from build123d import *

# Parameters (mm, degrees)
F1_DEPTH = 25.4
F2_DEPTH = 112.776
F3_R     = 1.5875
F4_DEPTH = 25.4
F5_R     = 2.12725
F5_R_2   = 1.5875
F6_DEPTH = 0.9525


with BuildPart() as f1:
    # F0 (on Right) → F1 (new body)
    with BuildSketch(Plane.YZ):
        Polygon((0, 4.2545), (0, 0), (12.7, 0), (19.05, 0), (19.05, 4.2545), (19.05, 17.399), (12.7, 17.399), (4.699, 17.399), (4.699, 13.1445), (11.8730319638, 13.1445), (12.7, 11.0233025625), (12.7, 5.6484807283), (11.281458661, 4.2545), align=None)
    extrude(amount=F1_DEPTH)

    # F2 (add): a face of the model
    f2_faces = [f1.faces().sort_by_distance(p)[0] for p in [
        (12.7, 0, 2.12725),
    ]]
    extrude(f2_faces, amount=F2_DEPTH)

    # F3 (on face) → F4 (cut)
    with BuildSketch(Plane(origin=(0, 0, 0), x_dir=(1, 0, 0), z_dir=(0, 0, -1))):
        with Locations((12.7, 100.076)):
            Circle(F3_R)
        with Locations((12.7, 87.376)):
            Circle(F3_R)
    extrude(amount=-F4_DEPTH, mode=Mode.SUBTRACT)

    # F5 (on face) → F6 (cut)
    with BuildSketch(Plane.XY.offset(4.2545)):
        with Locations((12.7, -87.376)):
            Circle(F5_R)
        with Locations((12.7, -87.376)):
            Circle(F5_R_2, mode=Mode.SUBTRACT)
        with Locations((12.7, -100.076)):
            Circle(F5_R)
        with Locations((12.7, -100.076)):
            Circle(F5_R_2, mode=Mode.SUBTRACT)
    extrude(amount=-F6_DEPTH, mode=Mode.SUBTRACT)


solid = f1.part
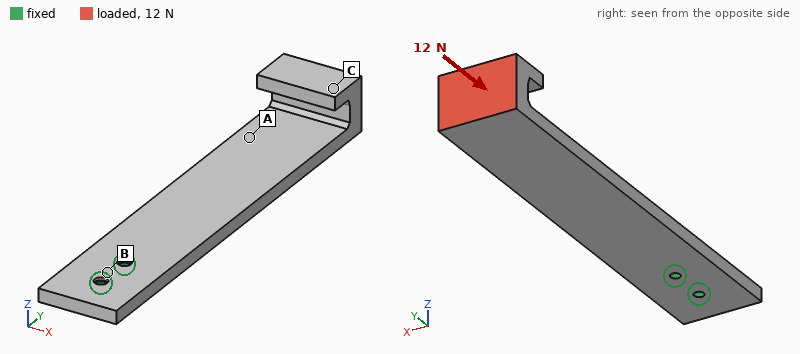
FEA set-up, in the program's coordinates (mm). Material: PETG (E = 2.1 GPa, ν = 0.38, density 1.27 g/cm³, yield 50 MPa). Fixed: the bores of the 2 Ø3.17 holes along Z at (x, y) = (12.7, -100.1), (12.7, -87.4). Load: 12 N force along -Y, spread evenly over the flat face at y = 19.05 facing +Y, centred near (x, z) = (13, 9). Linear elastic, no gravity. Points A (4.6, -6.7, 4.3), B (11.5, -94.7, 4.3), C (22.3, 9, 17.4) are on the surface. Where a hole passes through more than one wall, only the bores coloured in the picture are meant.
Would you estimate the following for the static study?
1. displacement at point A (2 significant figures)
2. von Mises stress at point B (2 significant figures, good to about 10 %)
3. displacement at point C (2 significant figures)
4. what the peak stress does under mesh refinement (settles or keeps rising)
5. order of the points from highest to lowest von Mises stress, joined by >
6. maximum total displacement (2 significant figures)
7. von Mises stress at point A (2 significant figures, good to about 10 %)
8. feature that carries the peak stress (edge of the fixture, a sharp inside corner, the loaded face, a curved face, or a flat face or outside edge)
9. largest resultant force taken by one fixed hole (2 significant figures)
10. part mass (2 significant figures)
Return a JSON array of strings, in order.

["0.78 mm", "0.30 MPa", "1.2 mm", "keeps rising", "A > B > C", "1.4 mm", "1.1 MPa", "edge of the fixture", "7.4 N", "22 g"]
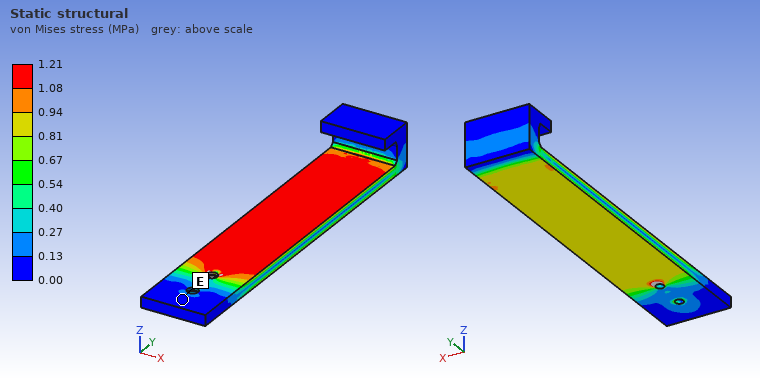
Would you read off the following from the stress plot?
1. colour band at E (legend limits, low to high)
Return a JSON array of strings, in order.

["0.00 to 0.13 MPa"]
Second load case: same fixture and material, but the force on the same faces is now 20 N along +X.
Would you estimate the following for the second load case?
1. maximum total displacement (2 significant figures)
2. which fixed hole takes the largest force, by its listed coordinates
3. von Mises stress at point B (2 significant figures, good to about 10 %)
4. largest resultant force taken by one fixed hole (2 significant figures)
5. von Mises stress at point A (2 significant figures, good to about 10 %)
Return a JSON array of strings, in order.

["1.5 mm", "(12.7, -87.4)", "1.5 MPa", "160 N", "2.0 MPa"]
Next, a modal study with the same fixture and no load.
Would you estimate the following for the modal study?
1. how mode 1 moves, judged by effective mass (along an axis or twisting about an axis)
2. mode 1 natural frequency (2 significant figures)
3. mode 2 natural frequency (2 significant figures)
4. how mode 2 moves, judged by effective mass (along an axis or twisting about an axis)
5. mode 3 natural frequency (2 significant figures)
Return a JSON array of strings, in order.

["along Z", "55 Hz", "240 Hz", "along X", "380 Hz"]
